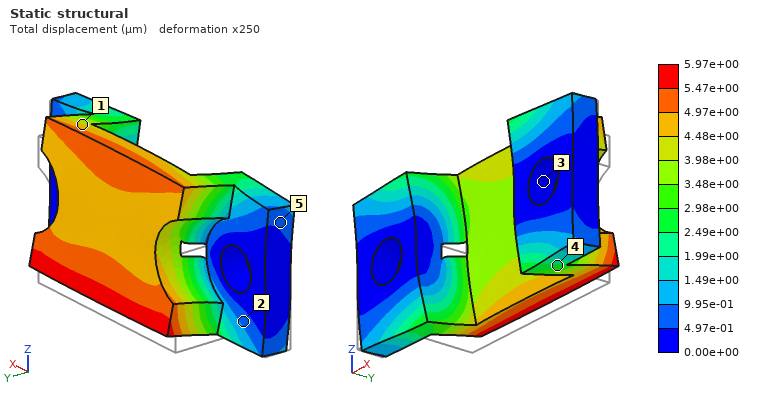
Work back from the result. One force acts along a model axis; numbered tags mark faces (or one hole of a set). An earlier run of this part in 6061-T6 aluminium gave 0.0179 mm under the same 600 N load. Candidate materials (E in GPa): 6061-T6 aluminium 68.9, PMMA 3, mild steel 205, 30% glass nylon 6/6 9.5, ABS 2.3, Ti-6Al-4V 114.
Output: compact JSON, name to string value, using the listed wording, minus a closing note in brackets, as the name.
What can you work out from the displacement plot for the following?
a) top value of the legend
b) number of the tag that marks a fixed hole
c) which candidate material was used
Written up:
{"top value of the legend": "5.97e+00 µm", "number of the tag that marks a fixed hole": "3", "which candidate material was used": "mild steel"}
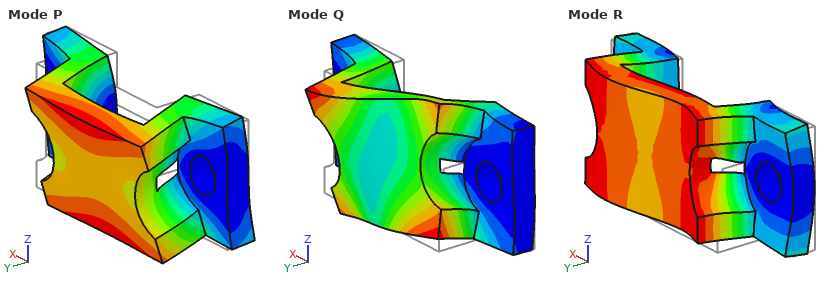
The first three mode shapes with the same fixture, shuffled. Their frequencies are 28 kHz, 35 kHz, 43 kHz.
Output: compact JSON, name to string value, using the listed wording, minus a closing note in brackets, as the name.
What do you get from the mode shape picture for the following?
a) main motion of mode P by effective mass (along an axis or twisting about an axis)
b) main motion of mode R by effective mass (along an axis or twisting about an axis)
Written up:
{"main motion of mode P by effective mass": "along Z", "main motion of mode R by effective mass": "along X"}
